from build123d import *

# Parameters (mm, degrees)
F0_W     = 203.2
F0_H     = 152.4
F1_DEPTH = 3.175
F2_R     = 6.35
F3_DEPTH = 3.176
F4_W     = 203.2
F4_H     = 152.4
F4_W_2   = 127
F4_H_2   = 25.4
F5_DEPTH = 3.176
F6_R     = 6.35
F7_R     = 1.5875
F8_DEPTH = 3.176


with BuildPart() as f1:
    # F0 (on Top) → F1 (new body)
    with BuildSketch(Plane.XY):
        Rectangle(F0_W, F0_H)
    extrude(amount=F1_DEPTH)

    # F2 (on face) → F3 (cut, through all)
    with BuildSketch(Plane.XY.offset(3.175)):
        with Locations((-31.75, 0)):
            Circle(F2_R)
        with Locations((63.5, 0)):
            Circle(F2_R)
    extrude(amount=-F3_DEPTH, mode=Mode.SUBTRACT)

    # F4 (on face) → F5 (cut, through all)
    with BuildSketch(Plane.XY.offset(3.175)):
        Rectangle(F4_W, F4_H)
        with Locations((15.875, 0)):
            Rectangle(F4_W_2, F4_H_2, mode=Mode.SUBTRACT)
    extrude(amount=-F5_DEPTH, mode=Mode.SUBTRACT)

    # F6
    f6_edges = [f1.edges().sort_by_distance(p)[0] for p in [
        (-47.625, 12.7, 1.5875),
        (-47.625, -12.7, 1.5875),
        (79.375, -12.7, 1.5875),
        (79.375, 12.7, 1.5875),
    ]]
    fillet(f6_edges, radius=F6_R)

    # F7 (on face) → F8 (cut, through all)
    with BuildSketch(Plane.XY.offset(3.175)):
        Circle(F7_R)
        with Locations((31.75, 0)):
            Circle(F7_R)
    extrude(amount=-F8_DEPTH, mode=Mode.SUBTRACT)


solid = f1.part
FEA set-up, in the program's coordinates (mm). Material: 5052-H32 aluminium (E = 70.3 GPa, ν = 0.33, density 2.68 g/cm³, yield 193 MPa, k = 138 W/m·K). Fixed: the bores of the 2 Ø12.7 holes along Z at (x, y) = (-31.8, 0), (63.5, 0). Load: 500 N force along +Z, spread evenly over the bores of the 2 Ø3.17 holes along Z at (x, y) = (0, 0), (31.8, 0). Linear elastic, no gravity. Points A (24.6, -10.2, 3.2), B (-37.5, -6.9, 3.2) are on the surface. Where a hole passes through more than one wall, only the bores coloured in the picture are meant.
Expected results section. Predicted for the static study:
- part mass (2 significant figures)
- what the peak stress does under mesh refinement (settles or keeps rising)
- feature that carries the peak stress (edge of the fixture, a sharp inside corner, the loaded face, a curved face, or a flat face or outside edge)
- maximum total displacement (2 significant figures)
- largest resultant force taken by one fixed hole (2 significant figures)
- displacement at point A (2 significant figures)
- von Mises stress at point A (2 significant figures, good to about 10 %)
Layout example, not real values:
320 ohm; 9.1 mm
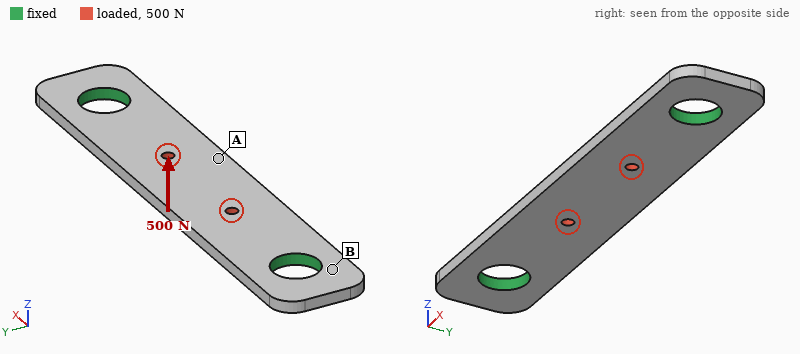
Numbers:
25 g; keeps rising; edge of the fixture; 0.23 mm; 250 N; 0.21 mm; 49 MPa
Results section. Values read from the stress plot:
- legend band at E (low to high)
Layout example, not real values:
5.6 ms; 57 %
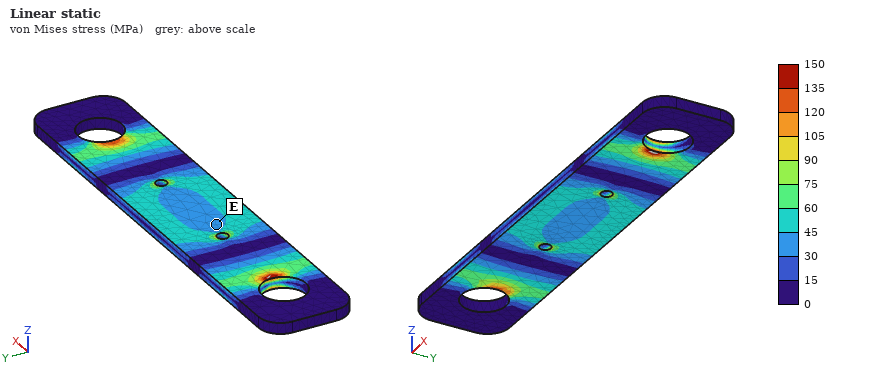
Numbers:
30 to 45 MPa
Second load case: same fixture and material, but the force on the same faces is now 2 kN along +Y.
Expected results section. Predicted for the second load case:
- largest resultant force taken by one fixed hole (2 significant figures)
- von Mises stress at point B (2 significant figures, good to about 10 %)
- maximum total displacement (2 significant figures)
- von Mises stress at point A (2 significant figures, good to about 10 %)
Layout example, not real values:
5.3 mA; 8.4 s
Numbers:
1.0 kN; 12 MPa; 39 µm; 27 MPa
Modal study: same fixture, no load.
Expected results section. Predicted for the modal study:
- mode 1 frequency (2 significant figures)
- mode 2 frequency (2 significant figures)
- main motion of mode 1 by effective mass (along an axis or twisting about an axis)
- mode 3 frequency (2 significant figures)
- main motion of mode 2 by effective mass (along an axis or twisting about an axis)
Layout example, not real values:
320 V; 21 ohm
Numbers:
2300 Hz; 4800 Hz; along Z; 6200 Hz; twisting about X
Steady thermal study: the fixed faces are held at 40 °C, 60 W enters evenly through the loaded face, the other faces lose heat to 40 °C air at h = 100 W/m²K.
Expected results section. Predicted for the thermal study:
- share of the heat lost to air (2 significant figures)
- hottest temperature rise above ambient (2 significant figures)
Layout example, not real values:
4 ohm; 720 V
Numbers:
30 %; 69 K
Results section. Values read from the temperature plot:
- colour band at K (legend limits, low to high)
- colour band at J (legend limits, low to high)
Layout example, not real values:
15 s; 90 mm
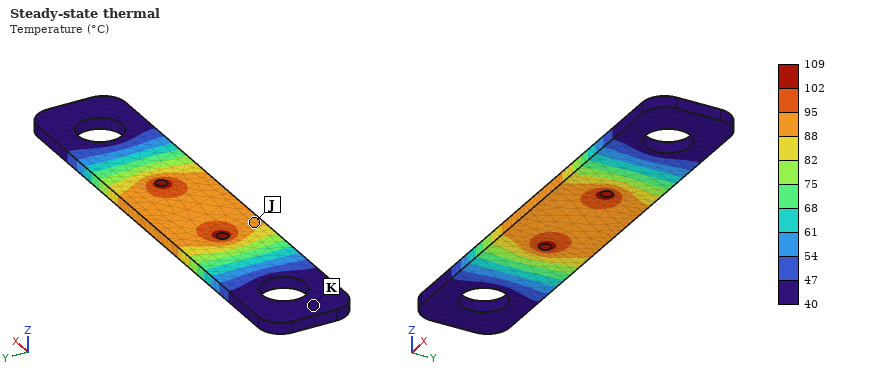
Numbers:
40 to 47 °C; 88 to 95 °C
